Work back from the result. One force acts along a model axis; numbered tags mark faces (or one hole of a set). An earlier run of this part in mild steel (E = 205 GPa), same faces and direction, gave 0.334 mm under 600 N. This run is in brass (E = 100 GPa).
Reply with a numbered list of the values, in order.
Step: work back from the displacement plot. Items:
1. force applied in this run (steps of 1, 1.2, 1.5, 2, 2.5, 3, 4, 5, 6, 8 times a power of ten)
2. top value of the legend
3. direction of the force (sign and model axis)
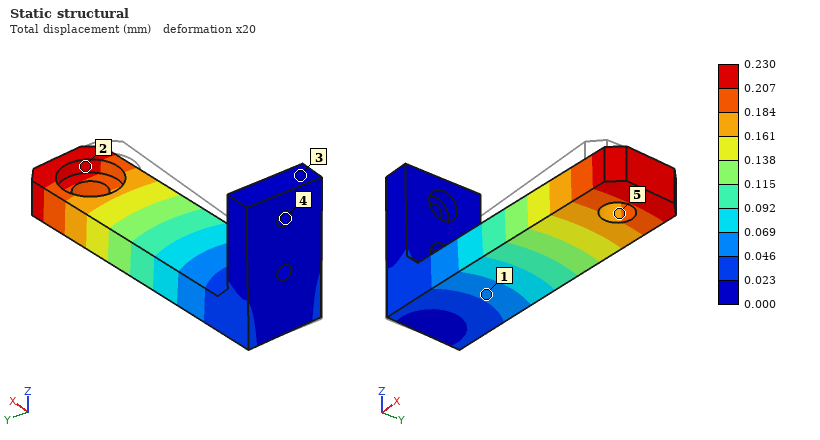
1. 200 N
2. 0.230 mm
3. +Y
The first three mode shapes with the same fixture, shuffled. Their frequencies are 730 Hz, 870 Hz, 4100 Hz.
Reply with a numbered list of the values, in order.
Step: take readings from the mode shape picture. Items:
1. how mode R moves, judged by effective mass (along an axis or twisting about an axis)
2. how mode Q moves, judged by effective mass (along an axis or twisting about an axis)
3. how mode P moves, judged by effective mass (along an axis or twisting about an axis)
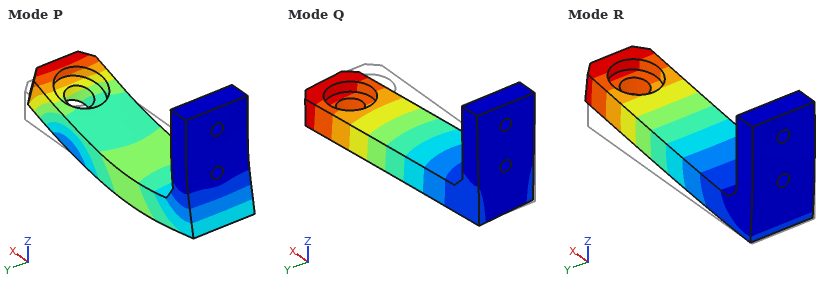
1. along Z
2. along Y
3. along X
